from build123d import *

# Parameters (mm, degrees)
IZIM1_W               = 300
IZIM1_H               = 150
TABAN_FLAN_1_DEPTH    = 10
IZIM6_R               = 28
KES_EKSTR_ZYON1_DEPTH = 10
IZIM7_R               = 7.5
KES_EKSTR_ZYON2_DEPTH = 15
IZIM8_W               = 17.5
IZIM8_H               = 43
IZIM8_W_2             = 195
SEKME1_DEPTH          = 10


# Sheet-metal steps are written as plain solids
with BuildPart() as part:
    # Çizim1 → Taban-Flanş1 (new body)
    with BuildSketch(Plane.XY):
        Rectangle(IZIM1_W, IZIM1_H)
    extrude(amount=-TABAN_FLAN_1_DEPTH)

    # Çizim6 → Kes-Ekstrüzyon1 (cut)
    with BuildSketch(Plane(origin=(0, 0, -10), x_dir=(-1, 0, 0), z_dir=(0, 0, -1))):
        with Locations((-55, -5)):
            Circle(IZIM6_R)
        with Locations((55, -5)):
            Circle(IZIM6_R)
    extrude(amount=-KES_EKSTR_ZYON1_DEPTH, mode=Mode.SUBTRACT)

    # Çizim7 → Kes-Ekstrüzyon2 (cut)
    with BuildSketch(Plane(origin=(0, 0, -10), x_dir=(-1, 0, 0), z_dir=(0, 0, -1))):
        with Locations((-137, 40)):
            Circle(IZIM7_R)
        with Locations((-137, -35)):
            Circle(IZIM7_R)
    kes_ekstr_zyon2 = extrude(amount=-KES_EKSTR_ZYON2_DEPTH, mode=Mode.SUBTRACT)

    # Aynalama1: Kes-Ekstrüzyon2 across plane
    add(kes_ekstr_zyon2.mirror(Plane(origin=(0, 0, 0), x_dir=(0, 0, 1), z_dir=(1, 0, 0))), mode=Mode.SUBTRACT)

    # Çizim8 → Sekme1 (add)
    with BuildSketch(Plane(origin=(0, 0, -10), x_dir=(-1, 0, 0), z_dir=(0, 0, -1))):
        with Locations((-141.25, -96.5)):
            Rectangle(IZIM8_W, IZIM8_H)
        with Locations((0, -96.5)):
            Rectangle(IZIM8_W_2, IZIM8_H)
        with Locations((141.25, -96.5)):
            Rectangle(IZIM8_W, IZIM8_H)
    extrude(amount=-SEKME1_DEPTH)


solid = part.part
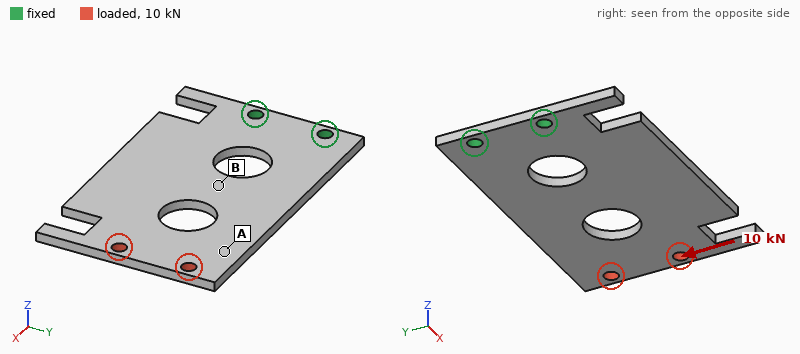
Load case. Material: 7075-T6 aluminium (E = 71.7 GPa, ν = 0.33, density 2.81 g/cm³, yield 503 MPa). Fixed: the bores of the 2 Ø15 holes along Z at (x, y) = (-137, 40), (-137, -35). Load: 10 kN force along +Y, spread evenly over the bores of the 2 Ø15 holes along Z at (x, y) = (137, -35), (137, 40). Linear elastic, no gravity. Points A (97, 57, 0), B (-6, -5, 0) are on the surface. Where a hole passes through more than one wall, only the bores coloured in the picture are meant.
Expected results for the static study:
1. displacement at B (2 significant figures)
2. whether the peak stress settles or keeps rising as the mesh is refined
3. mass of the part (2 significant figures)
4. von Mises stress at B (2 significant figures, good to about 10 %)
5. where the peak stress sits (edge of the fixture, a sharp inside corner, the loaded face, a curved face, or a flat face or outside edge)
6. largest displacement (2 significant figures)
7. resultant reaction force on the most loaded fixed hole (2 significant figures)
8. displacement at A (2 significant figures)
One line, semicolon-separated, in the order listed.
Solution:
0.27 mm; keeps rising; 1.4 kg; 39 MPa; edge of the fixture; 0.72 mm; 32 kN; 0.56 mm
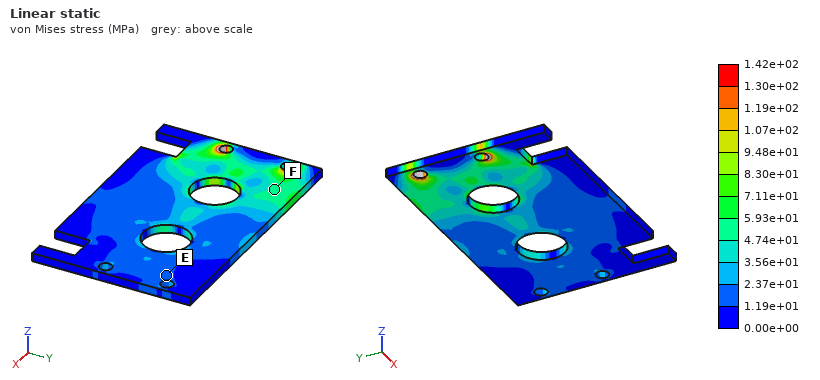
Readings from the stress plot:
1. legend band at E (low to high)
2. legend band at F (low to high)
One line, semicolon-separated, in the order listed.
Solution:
1.19e+01 to 2.37e+01 MPa; 4.74e+01 to 5.93e+01 MPa
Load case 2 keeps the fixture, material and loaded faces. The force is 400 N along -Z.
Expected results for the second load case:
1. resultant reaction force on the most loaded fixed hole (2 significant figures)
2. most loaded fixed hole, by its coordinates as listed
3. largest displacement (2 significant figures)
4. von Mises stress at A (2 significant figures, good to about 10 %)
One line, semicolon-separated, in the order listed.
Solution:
230 N; (-137, -35); 3.5 mm; 6.8 MPa
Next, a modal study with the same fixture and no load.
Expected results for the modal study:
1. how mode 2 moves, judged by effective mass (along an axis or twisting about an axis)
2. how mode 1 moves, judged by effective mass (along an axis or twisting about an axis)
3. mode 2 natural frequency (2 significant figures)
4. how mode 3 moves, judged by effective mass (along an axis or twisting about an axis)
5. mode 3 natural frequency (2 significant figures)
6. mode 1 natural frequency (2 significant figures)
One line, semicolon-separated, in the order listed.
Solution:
twisting about X; along Z; 290 Hz; along Z; 570 Hz; 92 Hz
